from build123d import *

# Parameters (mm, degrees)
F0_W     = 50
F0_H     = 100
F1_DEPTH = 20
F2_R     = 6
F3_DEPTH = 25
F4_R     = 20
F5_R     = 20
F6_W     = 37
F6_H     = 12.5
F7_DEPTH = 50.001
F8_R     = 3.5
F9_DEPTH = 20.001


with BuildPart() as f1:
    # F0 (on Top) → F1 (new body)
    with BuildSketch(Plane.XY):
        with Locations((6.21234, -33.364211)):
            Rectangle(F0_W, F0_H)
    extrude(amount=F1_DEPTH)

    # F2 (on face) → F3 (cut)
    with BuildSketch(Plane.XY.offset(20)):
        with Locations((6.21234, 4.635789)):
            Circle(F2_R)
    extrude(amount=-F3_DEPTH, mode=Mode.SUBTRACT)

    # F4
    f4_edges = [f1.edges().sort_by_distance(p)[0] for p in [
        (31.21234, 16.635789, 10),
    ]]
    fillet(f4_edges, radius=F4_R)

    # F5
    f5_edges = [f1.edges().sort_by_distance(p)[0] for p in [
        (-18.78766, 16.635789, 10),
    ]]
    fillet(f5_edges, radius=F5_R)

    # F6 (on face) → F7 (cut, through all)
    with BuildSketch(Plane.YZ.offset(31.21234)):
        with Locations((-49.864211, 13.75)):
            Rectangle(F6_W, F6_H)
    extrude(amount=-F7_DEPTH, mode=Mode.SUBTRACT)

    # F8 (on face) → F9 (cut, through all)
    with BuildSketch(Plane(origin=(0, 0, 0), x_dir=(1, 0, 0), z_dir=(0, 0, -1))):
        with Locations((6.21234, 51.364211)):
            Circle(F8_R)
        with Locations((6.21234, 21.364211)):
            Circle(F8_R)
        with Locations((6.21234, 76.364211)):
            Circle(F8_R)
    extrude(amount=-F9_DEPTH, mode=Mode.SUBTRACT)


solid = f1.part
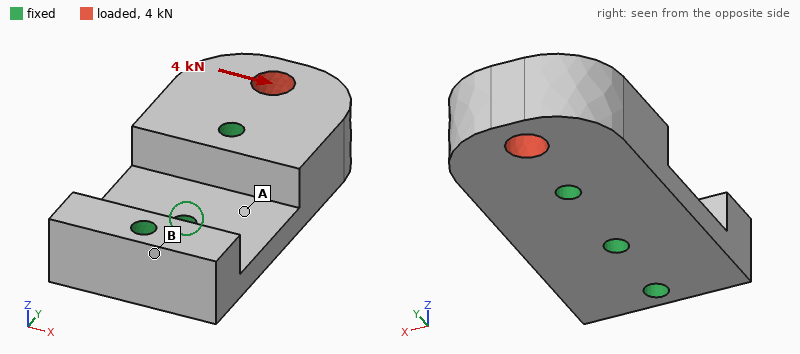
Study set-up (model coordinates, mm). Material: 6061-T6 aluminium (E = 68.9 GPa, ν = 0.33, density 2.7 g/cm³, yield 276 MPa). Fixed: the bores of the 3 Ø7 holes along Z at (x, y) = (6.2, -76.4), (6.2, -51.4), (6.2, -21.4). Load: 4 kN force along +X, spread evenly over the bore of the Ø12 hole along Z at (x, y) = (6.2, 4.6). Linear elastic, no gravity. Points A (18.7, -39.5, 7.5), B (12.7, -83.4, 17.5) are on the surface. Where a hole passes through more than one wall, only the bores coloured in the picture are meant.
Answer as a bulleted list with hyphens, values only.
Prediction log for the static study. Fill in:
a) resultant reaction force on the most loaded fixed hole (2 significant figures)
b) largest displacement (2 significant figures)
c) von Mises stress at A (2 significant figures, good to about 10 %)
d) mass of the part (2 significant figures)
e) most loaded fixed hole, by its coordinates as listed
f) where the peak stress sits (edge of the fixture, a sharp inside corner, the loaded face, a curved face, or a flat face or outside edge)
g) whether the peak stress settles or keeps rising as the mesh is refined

- 5.7 kN
- 25 µm
- 13 MPa
- 190 g
- (6.2, -21.4)
- edge of the fixture
- keeps rising
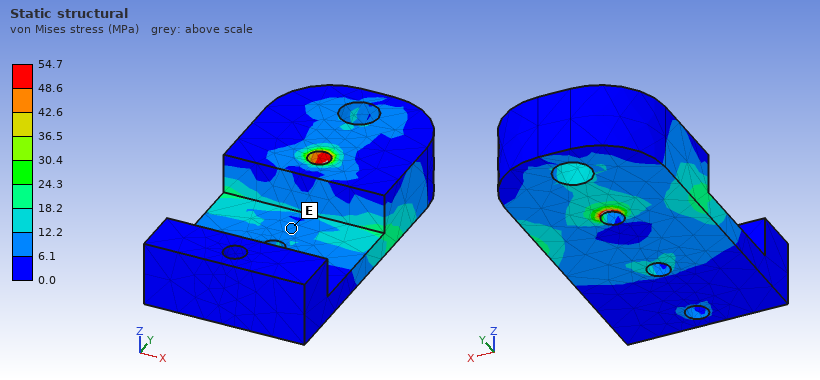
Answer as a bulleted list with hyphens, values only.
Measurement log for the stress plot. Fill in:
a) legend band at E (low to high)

- 6.1 to 12.2 MPa
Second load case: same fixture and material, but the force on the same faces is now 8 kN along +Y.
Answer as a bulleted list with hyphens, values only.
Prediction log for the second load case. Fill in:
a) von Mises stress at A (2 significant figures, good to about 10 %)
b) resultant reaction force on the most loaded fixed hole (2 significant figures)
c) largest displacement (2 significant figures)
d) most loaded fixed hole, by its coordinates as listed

- 5.2 MPa
- 6.9 kN
- 11 µm
- (6.2, -21.4)
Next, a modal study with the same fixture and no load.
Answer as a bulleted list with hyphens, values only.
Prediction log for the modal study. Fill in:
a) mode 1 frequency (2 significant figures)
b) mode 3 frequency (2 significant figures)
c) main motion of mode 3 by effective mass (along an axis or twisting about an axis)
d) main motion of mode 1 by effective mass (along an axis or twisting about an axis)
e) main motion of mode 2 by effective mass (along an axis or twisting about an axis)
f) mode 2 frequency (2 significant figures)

- 8800 Hz
- 12 kHz
- twisting about Y
- along Z
- along X
- 9300 Hz
